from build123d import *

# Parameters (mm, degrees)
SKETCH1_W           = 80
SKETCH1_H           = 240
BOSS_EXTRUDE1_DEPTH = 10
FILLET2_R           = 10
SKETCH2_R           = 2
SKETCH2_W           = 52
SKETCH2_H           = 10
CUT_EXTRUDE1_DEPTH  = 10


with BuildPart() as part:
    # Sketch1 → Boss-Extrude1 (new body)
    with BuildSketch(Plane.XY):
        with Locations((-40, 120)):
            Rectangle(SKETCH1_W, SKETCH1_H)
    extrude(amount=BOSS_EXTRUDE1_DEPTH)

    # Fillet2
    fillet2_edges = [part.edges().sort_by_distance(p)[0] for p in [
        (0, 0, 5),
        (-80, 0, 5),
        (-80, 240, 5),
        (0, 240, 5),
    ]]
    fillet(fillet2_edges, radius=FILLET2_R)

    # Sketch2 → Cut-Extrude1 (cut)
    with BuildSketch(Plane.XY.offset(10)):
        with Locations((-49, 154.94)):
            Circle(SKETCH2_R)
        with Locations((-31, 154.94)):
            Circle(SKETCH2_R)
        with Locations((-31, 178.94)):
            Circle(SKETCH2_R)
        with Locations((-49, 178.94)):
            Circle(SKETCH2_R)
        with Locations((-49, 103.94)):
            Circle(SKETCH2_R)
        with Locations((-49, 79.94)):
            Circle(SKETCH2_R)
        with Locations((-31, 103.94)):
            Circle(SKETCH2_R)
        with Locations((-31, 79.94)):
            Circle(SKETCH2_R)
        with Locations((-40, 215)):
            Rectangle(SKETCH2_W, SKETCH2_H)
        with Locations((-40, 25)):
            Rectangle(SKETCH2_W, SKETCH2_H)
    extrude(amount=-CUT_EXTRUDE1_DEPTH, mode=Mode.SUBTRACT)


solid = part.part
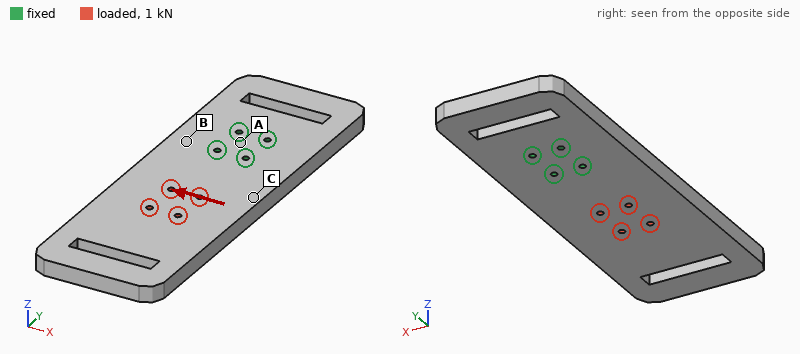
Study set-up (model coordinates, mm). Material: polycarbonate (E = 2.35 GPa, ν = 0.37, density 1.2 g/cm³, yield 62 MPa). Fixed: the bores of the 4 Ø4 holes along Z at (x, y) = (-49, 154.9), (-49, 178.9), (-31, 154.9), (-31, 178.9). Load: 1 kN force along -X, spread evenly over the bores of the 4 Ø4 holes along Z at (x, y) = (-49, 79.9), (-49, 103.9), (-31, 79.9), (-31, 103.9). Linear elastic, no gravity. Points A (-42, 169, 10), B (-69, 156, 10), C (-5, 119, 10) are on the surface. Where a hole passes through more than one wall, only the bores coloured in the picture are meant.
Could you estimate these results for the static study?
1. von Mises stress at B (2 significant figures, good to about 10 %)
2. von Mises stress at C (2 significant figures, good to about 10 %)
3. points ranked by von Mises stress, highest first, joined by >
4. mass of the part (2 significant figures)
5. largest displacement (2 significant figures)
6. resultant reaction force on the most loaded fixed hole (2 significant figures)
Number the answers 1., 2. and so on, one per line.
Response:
1. 3.8 MPa
2. 2.3 MPa
3. B > C > A
4. 220 g
5. 0.90 mm
6. 1.5 kN
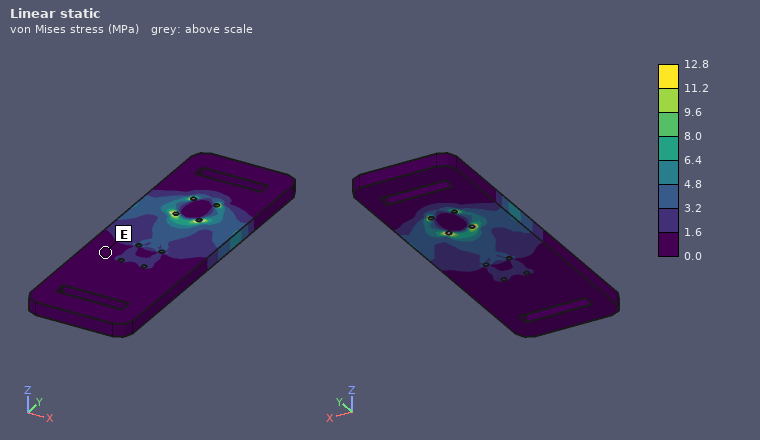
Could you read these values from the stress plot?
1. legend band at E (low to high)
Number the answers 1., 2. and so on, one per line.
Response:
1. 0.0 to 1.6 MPa
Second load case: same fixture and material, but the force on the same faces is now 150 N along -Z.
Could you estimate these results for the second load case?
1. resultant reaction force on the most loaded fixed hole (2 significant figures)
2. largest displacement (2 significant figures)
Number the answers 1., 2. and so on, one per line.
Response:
1. 160 N
2. 2.9 mm
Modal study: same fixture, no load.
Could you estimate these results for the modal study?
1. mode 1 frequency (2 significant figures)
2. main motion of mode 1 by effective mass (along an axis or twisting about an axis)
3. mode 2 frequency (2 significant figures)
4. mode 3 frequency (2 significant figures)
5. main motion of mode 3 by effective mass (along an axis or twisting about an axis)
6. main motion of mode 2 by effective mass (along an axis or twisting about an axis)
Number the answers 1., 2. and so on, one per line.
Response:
1. 97 Hz
2. along Z
3. 340 Hz
4. 460 Hz
5. along X
6. twisting about Y
